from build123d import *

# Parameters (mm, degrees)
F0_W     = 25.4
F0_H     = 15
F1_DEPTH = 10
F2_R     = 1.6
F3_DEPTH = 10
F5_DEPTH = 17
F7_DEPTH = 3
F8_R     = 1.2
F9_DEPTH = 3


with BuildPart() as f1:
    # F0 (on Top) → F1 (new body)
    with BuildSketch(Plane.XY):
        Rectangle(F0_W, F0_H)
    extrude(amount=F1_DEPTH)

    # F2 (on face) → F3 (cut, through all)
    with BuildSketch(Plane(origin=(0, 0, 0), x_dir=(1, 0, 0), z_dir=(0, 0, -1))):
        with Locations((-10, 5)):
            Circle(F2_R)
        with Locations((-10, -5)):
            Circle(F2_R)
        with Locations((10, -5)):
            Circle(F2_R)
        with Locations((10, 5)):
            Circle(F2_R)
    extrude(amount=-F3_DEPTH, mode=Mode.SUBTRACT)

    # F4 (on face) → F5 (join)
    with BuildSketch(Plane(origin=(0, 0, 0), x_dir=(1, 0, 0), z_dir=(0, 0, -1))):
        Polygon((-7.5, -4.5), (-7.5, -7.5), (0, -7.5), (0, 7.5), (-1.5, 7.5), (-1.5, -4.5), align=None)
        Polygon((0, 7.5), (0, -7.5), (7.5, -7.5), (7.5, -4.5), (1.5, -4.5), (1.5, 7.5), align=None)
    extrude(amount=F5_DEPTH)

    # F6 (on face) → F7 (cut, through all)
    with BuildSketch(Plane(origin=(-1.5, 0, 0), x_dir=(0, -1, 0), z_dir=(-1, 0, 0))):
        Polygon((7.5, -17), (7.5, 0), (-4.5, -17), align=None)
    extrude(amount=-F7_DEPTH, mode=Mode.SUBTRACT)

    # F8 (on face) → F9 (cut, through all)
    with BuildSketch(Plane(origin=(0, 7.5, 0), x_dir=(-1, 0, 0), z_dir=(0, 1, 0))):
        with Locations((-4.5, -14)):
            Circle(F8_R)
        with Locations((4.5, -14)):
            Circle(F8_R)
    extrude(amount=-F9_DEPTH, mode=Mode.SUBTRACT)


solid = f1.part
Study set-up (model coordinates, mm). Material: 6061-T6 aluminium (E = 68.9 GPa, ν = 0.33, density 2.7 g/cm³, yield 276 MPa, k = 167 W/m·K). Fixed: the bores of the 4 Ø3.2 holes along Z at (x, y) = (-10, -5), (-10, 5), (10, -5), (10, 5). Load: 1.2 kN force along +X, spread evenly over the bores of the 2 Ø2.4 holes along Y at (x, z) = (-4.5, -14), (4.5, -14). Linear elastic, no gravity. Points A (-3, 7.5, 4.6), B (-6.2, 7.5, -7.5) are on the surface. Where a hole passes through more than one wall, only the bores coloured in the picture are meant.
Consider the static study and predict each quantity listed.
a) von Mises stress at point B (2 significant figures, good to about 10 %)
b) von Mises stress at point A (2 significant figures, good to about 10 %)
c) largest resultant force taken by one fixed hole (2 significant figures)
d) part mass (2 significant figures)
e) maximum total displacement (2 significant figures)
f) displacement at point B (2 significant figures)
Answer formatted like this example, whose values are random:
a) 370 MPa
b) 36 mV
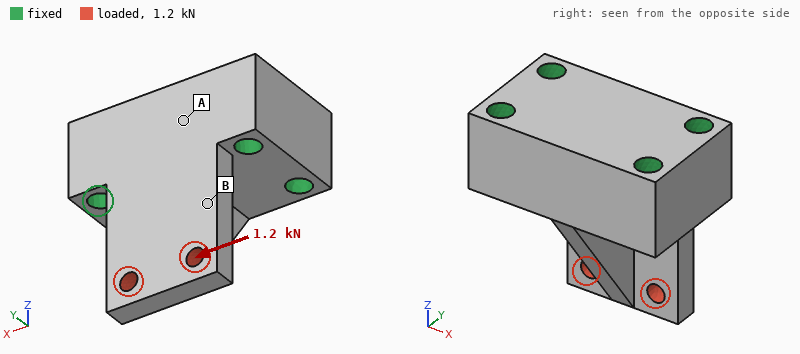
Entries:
a) 62 MPa
b) 23 MPa
c) 1.2 kN
d) 12 g
e) 60 µm
f) 26 µm
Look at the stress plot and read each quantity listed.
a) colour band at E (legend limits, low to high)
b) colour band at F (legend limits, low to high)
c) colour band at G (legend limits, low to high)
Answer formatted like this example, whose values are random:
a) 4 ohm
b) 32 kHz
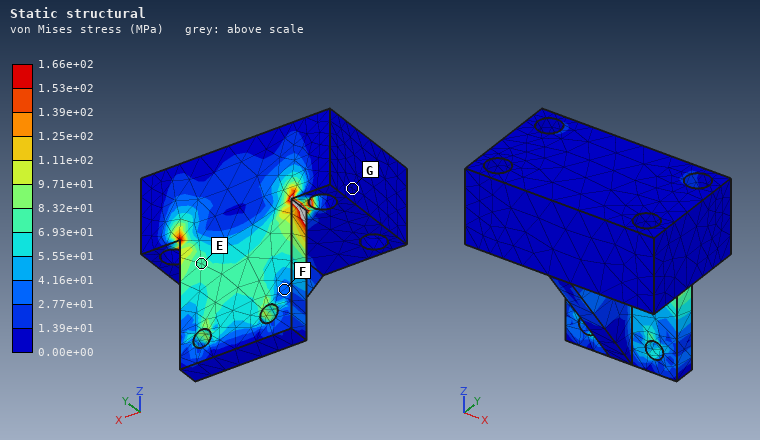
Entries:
a) 6.93e+01 to 8.32e+01 MPa
b) 2.77e+01 to 4.16e+01 MPa
c) 0.00e+00 to 1.39e+01 MPa
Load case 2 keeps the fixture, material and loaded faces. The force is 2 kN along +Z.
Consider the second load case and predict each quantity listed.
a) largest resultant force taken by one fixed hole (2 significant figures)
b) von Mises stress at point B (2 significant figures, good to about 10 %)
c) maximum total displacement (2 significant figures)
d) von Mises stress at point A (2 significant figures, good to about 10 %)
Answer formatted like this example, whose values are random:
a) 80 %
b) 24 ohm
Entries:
a) 980 N
b) 53 MPa
c) 26 µm
d) 22 MPa
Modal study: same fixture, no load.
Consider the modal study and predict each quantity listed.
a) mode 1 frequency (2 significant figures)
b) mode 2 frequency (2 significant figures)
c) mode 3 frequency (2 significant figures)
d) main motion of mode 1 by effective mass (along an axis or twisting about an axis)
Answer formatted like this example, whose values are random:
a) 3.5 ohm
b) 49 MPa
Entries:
a) 19 kHz
b) 23 kHz
c) 24 kHz
d) along Y
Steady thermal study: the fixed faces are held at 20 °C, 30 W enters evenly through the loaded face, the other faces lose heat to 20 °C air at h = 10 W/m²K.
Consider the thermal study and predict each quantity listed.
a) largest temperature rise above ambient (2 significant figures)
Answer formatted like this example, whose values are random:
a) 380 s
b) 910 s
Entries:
a) 58 K
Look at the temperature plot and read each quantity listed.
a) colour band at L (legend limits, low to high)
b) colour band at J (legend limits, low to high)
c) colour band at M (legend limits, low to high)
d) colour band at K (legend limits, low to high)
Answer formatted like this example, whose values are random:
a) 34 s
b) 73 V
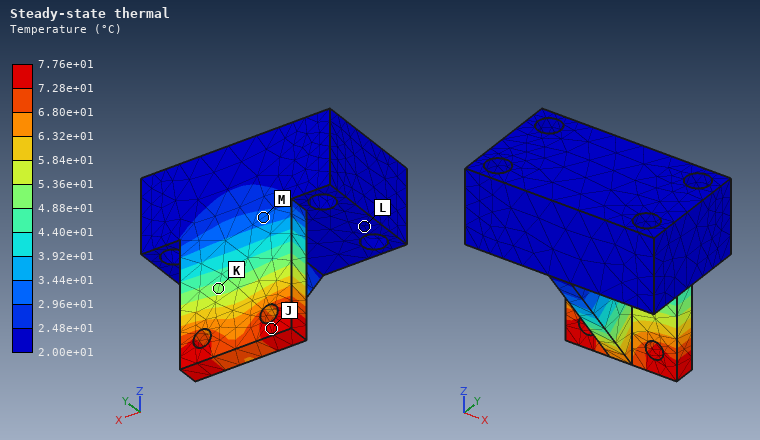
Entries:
a) 2.00e+01 to 2.48e+01 °C
b) 7.28e+01 to 7.76e+01 °C
c) 2.96e+01 to 3.44e+01 °C
d) 4.88e+01 to 5.36e+01 °C
